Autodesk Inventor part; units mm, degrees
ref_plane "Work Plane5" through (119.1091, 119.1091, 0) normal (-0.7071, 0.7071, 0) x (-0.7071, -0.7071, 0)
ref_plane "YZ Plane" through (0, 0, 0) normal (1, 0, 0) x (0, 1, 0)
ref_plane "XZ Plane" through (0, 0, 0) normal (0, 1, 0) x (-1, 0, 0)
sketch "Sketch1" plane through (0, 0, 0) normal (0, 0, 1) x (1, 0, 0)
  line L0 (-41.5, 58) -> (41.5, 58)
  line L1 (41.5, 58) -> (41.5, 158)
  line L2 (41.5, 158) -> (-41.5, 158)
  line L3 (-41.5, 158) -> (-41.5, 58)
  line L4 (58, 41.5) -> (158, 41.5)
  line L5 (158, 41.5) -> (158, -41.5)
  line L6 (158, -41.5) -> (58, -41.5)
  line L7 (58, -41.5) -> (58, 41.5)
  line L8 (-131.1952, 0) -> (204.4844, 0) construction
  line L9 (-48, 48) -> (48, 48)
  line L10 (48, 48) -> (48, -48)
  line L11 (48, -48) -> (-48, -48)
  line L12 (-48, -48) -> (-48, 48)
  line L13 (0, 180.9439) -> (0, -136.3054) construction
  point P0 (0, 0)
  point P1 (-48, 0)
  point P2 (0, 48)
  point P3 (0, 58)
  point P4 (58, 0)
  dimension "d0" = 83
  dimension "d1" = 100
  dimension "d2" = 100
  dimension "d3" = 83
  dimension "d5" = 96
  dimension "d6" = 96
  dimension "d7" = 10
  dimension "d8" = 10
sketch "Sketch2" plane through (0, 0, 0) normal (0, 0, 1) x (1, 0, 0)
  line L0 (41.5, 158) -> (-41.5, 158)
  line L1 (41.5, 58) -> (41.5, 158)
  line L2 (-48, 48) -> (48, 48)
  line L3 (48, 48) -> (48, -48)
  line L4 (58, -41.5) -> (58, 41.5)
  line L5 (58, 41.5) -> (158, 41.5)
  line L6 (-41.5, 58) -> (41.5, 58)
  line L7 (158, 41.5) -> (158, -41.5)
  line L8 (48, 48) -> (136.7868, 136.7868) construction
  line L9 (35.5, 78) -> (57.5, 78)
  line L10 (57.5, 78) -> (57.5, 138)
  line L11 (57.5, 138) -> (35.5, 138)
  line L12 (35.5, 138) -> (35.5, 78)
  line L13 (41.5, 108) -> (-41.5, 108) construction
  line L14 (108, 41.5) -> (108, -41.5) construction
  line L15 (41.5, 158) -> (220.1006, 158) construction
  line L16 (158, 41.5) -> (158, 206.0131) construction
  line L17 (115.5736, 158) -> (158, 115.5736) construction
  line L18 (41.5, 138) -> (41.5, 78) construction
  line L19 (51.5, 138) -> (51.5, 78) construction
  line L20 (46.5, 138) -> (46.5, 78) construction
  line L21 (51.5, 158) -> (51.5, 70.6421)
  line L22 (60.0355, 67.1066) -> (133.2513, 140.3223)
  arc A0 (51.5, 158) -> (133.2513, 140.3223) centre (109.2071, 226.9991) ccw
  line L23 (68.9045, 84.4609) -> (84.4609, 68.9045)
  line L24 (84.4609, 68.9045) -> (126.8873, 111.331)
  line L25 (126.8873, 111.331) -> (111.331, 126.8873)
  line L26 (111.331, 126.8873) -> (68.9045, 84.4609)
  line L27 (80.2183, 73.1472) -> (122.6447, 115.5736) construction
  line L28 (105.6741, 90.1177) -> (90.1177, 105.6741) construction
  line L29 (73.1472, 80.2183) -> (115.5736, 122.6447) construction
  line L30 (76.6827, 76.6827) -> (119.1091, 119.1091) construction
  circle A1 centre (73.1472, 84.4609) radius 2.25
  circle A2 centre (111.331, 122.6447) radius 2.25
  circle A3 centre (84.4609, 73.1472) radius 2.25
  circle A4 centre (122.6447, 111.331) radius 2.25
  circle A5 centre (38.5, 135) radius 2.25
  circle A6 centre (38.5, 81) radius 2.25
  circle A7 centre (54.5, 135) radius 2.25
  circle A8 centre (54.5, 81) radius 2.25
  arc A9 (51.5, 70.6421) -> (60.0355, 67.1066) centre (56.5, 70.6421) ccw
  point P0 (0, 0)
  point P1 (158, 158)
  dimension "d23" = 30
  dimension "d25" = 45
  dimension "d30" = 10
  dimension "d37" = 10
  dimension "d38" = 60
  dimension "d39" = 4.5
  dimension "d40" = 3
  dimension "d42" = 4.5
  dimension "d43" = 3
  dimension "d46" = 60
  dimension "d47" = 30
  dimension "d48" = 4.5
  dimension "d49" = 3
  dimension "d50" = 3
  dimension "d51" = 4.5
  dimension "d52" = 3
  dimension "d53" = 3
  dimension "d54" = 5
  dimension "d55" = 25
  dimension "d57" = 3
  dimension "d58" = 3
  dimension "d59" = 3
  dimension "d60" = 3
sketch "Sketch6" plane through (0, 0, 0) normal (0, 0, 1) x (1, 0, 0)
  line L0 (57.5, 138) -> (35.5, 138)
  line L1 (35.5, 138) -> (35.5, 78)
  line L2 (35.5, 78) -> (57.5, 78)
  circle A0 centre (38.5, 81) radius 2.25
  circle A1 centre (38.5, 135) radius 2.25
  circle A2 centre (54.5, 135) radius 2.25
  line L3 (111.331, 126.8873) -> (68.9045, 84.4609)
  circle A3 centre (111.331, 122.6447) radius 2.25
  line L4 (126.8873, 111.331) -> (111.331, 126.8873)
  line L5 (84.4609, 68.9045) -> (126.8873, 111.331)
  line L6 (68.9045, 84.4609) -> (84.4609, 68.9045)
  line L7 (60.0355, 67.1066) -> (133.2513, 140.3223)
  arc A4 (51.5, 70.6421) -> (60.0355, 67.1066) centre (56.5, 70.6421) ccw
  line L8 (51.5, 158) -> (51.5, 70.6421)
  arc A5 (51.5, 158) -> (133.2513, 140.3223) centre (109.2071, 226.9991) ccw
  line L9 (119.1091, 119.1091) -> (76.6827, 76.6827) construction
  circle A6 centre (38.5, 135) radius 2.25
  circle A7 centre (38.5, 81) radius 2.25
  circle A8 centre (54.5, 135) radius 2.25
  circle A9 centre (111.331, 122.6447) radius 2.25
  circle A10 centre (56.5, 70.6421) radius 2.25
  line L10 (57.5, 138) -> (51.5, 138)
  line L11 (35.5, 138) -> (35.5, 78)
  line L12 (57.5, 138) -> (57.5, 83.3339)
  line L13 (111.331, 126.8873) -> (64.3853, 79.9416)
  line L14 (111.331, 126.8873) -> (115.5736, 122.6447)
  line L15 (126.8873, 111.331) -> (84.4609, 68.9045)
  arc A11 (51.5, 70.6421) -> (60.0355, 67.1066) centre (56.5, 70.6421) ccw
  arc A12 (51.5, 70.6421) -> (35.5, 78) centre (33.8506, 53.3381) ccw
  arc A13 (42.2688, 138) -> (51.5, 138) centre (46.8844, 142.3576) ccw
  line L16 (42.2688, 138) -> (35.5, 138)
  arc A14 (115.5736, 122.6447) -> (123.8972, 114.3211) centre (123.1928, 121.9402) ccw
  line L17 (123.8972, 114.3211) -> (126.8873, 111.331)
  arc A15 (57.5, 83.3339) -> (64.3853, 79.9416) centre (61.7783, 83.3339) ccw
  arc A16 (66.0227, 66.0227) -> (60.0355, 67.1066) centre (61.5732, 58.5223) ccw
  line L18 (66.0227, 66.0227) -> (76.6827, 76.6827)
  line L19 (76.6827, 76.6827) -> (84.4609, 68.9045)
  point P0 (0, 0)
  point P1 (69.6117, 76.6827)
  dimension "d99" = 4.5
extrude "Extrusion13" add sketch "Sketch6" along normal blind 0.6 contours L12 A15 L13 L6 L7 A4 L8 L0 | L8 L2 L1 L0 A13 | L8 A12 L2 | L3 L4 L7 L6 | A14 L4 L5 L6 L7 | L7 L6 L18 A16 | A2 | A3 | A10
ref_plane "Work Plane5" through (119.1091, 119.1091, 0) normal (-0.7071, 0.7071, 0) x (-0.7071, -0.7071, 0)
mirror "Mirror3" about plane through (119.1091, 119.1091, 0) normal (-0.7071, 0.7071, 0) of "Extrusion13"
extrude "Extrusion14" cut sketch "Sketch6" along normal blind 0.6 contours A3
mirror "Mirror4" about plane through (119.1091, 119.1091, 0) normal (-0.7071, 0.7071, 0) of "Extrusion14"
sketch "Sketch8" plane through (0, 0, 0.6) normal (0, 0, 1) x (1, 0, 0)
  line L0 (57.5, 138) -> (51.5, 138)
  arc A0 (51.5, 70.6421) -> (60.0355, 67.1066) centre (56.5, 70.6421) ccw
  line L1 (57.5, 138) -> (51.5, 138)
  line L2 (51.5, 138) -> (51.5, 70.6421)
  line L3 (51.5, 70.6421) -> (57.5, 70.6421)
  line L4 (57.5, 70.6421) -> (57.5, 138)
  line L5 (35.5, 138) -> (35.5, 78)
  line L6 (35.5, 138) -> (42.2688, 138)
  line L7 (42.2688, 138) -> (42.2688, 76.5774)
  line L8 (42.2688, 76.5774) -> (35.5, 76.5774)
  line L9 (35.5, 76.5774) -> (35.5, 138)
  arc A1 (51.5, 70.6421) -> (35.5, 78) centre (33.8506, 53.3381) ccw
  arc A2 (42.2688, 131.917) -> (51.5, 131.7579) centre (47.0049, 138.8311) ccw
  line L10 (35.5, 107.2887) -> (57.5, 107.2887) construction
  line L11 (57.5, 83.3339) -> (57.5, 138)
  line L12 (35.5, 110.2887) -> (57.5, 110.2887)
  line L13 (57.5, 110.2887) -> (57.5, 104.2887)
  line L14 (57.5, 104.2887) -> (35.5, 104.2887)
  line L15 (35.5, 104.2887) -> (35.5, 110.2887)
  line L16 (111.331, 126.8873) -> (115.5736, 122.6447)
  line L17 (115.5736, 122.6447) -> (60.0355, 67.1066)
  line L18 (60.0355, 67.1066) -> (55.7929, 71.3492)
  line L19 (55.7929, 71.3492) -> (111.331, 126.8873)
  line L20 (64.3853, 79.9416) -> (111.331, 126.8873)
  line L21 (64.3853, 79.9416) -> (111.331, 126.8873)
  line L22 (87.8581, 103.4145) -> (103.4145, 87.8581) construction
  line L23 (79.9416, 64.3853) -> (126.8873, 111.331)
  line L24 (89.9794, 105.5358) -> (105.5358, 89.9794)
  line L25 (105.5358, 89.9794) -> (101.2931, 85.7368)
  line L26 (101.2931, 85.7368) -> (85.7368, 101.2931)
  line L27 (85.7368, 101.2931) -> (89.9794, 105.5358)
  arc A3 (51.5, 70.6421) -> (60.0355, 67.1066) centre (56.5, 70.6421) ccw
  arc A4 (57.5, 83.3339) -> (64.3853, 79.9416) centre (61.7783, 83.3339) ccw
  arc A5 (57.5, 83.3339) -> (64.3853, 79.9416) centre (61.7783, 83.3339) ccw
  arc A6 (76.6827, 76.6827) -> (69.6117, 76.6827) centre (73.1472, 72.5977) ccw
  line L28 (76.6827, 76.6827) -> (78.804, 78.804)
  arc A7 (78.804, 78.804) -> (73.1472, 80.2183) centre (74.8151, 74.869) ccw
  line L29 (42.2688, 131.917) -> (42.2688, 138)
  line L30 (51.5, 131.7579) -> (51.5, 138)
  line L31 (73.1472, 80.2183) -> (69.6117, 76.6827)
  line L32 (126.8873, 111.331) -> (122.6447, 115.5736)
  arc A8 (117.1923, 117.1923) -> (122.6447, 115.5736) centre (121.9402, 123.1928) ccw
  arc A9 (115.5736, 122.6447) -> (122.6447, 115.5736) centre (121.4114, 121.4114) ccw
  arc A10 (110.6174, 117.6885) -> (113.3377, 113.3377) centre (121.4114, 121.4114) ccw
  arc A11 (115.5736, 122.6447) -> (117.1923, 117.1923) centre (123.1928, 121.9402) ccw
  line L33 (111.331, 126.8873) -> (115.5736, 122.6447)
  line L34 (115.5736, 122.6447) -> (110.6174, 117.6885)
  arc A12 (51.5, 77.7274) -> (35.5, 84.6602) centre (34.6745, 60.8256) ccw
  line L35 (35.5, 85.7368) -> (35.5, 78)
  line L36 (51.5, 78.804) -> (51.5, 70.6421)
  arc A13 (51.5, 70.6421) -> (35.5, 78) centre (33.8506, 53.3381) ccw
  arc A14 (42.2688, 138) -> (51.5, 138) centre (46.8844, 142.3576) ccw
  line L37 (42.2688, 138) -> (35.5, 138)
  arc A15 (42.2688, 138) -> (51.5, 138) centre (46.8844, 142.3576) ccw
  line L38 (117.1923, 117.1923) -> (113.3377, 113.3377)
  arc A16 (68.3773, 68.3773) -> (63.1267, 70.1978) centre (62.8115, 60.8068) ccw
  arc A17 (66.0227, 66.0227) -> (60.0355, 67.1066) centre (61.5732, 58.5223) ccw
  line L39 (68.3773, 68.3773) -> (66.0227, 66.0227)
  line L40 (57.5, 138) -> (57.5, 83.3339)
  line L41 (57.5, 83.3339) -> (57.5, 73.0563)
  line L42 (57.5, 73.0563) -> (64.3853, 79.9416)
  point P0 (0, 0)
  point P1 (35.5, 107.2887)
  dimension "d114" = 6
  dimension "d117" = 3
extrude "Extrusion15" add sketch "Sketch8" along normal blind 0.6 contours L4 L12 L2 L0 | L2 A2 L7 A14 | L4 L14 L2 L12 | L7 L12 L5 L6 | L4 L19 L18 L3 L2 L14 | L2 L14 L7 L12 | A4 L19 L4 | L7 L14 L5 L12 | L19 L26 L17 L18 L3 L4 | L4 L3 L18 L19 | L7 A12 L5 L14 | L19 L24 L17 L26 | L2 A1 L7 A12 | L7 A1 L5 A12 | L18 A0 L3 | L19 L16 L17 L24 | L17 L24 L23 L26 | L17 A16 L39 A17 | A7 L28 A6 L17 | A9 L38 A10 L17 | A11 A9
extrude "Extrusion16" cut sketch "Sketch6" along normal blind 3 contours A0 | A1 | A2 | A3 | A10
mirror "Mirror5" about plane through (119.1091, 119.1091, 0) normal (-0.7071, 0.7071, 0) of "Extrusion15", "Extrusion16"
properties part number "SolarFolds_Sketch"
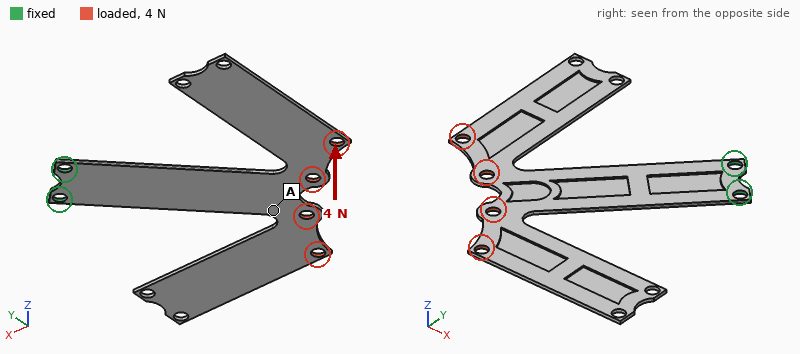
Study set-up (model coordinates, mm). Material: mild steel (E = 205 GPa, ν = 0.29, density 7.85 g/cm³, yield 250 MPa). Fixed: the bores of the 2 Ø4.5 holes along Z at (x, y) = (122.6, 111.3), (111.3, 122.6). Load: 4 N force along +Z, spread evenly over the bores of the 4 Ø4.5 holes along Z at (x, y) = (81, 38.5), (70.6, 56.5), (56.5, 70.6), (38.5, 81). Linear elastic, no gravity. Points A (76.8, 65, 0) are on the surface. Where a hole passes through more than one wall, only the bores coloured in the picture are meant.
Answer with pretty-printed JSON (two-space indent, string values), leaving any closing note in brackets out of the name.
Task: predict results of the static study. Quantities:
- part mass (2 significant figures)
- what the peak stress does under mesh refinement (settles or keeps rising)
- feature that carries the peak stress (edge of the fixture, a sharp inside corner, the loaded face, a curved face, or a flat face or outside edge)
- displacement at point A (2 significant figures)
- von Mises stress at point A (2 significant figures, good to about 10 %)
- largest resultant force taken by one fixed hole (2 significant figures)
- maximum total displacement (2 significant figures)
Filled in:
{
  "part mass": "35 g",
  "what the peak stress does under mesh refinement": "keeps rising",
  "feature that carries the peak stress": "edge of the fixture",
  "displacement at point A": "0.92 mm",
  "von Mises stress at point A": "14 MPa",
  "largest resultant force taken by one fixed hole": "33 N",
  "maximum total displacement": "1.4 mm"
}
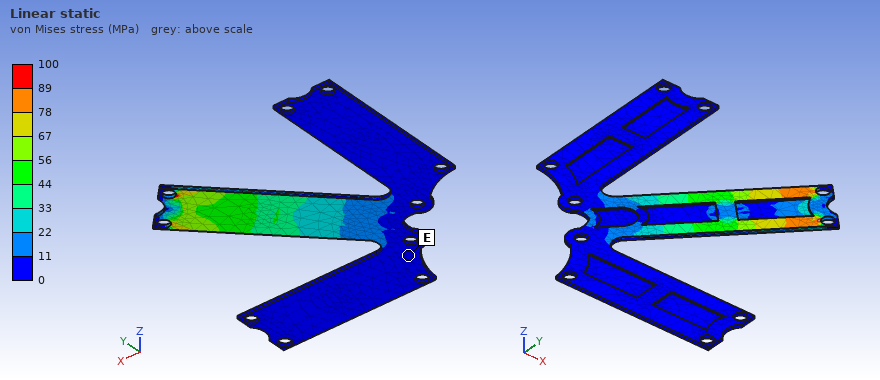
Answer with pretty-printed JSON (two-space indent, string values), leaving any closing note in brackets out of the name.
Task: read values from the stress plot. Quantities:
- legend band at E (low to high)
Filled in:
{
  "legend band at E": "0 to 11 MPa"
}
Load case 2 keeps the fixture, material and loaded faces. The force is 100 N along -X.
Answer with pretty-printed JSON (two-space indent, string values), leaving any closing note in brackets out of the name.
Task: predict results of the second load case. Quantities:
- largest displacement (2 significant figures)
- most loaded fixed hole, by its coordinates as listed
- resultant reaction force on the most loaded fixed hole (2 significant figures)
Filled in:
{
  "largest displacement": "0.18 mm",
  "most loaded fixed hole, by its coordinates as listed": "(122.6, 111.3)",
  "resultant reaction force on the most loaded fixed hole": "360 N"
}
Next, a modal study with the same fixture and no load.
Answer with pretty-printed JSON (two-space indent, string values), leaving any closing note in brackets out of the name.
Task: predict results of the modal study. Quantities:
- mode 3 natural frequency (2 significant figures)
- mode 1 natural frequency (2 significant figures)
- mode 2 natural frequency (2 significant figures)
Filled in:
{
  "mode 3 natural frequency": "170 Hz",
  "mode 1 natural frequency": "76 Hz",
  "mode 2 natural frequency": "76 Hz"
}
